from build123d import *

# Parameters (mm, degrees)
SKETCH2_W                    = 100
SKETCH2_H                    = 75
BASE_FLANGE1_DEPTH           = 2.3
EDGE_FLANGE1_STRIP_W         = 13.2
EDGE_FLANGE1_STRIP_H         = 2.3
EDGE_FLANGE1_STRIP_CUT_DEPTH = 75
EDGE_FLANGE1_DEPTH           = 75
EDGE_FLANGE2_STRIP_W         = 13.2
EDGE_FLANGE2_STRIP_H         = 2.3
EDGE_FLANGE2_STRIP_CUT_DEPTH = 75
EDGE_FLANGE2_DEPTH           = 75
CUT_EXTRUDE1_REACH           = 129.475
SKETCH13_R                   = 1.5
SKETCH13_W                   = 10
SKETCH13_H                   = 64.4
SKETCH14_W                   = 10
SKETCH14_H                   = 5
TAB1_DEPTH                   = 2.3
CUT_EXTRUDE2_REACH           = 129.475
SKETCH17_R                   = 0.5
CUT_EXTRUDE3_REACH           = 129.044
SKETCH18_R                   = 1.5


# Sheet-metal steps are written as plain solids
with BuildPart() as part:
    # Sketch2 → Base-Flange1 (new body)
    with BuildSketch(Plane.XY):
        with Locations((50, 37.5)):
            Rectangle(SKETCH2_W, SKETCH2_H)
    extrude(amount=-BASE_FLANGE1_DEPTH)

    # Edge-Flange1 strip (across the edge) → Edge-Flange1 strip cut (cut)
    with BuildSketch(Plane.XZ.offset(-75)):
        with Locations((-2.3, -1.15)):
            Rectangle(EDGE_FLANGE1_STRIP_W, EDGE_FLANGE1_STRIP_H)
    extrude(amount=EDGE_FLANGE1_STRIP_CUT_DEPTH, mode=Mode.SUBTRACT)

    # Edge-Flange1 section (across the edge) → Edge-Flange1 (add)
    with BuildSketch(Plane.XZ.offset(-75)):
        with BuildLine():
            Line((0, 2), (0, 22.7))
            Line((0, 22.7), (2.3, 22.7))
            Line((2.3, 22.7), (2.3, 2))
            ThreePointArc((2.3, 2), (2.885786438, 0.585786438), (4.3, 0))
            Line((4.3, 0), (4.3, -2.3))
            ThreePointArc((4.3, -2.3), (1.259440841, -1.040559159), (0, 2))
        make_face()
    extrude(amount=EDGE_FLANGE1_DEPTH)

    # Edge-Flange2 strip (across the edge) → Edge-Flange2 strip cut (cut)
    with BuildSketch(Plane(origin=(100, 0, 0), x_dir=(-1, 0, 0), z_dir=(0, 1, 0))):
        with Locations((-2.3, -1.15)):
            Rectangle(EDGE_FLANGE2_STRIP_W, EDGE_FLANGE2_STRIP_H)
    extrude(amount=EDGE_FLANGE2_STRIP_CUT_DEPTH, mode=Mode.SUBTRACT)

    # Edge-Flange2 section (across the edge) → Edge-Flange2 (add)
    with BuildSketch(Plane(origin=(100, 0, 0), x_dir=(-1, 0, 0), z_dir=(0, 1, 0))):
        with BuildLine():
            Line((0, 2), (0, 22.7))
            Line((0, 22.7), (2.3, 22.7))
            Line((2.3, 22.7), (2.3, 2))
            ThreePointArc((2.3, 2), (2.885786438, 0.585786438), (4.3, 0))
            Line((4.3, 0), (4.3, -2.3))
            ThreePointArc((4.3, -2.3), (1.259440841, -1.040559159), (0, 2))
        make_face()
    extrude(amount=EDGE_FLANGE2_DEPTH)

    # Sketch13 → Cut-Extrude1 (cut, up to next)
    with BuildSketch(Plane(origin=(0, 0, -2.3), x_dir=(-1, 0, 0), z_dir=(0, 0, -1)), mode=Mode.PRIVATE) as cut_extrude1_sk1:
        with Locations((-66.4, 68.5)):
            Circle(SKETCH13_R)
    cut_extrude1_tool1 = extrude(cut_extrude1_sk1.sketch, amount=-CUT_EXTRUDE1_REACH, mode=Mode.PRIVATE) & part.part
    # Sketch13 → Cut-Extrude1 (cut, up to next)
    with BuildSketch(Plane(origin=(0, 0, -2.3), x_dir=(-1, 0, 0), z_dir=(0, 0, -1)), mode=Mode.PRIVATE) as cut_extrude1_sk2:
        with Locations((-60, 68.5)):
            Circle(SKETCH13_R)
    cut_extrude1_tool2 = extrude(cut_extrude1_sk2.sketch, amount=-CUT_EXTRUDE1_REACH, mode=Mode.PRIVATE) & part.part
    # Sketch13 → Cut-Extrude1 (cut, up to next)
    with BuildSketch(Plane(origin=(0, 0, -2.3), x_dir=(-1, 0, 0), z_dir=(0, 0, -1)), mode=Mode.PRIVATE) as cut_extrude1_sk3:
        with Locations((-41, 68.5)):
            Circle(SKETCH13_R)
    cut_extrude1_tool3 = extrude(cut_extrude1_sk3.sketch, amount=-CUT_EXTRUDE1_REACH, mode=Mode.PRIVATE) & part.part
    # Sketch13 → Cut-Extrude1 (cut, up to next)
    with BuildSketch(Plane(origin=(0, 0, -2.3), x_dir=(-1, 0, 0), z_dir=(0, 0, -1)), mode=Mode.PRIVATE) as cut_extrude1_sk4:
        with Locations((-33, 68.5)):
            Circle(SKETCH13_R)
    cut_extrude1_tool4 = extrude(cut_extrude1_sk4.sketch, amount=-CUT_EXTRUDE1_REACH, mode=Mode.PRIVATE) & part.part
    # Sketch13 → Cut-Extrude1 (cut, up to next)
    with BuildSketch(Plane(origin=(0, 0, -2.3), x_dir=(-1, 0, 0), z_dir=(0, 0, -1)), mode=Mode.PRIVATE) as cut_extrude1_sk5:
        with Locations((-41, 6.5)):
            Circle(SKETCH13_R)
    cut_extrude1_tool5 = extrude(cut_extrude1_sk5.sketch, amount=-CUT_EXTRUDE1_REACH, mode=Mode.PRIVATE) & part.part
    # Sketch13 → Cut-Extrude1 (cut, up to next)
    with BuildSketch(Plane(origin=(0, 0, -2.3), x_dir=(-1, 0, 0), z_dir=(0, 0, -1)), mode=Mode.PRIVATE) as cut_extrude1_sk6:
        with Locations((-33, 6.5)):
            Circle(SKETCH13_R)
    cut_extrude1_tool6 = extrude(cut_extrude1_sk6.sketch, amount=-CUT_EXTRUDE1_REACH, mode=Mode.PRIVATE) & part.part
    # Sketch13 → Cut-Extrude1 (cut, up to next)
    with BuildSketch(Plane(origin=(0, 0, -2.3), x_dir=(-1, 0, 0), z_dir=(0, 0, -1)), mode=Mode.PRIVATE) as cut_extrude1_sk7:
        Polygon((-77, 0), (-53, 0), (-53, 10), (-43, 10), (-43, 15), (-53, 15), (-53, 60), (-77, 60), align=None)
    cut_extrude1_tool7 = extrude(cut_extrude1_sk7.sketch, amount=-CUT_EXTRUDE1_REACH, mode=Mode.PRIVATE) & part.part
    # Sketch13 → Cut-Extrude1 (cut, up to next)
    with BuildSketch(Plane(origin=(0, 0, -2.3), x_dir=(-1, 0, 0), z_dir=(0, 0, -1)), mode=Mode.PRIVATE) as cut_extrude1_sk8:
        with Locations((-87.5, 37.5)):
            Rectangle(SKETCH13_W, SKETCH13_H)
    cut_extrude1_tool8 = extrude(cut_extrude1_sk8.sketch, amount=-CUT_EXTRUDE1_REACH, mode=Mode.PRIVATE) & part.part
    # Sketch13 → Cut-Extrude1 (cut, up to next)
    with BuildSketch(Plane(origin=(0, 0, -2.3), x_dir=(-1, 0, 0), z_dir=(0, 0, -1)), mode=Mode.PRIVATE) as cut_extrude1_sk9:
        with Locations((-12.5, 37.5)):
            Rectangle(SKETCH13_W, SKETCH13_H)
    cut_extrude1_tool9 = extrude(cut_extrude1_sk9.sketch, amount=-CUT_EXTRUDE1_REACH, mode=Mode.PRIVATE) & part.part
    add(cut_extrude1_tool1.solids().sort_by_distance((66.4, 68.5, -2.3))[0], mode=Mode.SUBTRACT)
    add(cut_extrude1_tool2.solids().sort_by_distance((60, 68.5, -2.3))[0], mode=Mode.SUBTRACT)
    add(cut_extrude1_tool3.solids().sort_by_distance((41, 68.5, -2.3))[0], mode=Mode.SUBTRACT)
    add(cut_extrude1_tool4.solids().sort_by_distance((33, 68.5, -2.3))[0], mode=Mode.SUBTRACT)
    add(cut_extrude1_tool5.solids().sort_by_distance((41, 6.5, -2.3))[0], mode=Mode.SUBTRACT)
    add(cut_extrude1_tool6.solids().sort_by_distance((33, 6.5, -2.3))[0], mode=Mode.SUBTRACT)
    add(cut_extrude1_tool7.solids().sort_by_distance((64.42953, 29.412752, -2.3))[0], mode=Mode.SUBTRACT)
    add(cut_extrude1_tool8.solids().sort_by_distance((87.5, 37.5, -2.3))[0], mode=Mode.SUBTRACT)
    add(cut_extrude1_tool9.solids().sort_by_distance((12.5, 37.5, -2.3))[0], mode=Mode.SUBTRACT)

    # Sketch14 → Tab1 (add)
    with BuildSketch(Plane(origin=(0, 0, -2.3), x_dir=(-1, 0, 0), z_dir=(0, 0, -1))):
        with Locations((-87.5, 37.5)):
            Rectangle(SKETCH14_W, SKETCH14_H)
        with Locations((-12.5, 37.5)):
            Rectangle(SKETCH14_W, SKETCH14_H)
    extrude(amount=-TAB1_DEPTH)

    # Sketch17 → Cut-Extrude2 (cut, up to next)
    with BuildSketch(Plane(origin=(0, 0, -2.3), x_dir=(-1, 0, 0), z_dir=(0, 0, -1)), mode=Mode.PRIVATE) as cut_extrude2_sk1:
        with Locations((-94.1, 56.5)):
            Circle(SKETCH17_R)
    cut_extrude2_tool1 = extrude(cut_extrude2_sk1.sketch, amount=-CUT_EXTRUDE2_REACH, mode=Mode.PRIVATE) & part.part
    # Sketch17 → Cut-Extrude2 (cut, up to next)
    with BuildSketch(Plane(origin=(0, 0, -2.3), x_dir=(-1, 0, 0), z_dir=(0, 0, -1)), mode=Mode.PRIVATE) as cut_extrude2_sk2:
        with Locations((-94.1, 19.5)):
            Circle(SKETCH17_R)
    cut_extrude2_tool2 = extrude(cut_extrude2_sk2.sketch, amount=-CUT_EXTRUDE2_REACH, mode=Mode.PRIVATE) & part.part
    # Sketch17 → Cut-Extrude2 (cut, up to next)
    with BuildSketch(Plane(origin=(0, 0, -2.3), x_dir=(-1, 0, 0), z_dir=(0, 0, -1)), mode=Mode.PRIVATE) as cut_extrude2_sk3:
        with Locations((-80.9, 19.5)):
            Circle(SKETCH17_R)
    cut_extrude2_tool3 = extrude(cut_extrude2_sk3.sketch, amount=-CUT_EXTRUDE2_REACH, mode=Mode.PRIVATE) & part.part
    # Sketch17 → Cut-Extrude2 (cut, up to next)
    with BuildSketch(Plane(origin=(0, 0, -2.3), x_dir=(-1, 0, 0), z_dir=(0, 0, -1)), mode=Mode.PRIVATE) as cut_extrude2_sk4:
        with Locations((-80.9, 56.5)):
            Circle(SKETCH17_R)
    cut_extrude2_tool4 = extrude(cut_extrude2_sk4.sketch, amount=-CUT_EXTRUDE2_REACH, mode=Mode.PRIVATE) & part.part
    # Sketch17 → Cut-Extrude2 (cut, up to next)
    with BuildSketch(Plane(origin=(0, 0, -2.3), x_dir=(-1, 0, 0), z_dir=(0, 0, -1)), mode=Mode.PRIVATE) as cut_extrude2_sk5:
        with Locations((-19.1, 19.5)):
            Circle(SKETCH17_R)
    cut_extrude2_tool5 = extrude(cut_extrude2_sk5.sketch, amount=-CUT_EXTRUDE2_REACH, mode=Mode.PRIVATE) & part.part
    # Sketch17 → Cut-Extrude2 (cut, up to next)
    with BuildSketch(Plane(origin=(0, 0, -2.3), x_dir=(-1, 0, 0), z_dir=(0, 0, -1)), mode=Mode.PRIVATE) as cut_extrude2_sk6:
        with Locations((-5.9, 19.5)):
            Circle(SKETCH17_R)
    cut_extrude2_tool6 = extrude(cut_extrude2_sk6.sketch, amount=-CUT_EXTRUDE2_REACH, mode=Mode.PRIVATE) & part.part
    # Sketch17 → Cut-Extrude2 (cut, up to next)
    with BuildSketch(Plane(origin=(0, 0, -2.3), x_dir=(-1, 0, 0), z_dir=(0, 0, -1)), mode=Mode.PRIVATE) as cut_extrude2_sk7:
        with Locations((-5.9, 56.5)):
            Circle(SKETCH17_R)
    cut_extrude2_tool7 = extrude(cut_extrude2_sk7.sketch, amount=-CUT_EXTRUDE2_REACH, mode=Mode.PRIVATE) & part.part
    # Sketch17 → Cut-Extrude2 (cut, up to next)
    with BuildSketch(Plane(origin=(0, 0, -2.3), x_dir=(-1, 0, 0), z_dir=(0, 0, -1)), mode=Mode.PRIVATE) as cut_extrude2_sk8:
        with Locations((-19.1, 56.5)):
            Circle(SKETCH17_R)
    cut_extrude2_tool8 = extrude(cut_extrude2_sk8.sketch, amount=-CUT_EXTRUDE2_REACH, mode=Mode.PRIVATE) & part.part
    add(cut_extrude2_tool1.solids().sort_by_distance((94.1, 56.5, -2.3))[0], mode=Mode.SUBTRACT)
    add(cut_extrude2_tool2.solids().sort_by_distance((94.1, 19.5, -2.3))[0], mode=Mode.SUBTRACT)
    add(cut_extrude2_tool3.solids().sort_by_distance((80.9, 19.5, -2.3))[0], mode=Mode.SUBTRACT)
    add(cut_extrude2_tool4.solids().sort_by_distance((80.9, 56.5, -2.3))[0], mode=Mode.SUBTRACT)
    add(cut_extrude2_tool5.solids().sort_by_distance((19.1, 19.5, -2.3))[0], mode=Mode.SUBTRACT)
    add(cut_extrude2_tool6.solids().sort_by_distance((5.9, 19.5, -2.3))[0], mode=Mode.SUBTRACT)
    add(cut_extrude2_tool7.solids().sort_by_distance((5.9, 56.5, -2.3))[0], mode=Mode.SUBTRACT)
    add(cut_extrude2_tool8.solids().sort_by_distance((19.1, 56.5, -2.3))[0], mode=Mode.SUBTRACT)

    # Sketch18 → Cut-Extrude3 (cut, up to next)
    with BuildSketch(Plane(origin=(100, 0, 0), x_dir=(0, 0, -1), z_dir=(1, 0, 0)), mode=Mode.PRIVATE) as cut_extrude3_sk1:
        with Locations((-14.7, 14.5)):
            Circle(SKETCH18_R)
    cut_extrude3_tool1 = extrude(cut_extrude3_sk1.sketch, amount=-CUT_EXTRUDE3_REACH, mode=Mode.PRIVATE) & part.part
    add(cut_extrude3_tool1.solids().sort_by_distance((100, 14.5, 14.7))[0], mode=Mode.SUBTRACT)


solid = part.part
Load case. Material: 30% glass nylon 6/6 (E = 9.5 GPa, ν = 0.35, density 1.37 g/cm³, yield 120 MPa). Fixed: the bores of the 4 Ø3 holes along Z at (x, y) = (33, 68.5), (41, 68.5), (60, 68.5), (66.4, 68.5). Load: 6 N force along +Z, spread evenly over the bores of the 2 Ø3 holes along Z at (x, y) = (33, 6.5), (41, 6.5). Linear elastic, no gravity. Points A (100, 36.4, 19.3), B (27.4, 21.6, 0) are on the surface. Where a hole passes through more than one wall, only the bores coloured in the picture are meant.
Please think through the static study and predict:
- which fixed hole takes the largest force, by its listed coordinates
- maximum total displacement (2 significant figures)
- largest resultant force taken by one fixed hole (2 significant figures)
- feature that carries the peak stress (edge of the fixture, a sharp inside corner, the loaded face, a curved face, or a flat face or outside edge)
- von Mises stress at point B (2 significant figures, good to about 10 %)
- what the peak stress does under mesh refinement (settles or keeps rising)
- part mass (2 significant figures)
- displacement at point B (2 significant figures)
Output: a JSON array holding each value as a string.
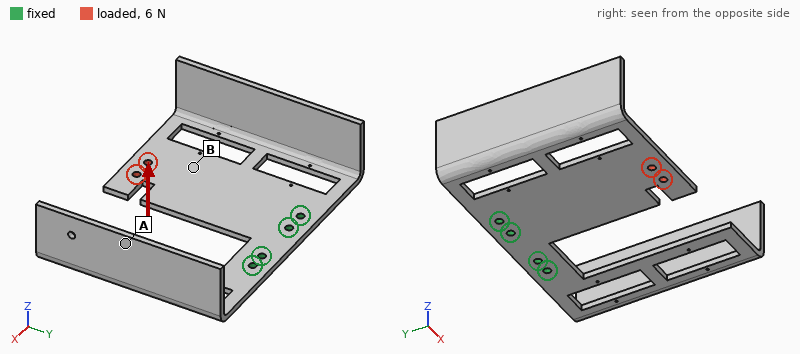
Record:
["(41, 68.5)", "1.2 mm", "6.1 N", "edge of the fixture", "2.4 MPa", "keeps rising", "25 g", "0.68 mm"]
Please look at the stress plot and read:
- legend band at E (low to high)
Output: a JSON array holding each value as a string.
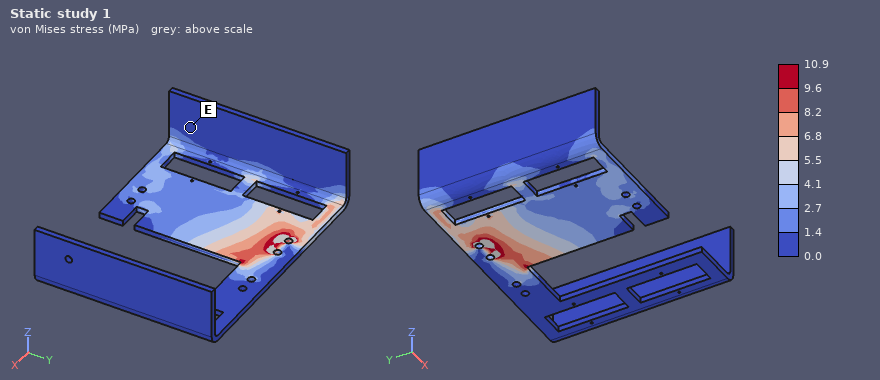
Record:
["0.0 to 1.4 MPa"]
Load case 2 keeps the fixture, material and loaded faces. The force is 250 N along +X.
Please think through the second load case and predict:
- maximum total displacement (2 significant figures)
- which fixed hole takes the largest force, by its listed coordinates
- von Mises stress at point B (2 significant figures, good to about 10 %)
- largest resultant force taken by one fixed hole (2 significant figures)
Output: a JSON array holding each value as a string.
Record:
["0.61 mm", "(33, 68.5)", "6.9 MPa", "810 N"]
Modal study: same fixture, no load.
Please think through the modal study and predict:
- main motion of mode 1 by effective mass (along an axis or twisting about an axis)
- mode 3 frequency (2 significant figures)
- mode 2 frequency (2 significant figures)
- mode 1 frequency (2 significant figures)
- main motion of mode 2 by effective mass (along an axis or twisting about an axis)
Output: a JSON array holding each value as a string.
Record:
["along Z", "230 Hz", "150 Hz", "100 Hz", "along Z"]
